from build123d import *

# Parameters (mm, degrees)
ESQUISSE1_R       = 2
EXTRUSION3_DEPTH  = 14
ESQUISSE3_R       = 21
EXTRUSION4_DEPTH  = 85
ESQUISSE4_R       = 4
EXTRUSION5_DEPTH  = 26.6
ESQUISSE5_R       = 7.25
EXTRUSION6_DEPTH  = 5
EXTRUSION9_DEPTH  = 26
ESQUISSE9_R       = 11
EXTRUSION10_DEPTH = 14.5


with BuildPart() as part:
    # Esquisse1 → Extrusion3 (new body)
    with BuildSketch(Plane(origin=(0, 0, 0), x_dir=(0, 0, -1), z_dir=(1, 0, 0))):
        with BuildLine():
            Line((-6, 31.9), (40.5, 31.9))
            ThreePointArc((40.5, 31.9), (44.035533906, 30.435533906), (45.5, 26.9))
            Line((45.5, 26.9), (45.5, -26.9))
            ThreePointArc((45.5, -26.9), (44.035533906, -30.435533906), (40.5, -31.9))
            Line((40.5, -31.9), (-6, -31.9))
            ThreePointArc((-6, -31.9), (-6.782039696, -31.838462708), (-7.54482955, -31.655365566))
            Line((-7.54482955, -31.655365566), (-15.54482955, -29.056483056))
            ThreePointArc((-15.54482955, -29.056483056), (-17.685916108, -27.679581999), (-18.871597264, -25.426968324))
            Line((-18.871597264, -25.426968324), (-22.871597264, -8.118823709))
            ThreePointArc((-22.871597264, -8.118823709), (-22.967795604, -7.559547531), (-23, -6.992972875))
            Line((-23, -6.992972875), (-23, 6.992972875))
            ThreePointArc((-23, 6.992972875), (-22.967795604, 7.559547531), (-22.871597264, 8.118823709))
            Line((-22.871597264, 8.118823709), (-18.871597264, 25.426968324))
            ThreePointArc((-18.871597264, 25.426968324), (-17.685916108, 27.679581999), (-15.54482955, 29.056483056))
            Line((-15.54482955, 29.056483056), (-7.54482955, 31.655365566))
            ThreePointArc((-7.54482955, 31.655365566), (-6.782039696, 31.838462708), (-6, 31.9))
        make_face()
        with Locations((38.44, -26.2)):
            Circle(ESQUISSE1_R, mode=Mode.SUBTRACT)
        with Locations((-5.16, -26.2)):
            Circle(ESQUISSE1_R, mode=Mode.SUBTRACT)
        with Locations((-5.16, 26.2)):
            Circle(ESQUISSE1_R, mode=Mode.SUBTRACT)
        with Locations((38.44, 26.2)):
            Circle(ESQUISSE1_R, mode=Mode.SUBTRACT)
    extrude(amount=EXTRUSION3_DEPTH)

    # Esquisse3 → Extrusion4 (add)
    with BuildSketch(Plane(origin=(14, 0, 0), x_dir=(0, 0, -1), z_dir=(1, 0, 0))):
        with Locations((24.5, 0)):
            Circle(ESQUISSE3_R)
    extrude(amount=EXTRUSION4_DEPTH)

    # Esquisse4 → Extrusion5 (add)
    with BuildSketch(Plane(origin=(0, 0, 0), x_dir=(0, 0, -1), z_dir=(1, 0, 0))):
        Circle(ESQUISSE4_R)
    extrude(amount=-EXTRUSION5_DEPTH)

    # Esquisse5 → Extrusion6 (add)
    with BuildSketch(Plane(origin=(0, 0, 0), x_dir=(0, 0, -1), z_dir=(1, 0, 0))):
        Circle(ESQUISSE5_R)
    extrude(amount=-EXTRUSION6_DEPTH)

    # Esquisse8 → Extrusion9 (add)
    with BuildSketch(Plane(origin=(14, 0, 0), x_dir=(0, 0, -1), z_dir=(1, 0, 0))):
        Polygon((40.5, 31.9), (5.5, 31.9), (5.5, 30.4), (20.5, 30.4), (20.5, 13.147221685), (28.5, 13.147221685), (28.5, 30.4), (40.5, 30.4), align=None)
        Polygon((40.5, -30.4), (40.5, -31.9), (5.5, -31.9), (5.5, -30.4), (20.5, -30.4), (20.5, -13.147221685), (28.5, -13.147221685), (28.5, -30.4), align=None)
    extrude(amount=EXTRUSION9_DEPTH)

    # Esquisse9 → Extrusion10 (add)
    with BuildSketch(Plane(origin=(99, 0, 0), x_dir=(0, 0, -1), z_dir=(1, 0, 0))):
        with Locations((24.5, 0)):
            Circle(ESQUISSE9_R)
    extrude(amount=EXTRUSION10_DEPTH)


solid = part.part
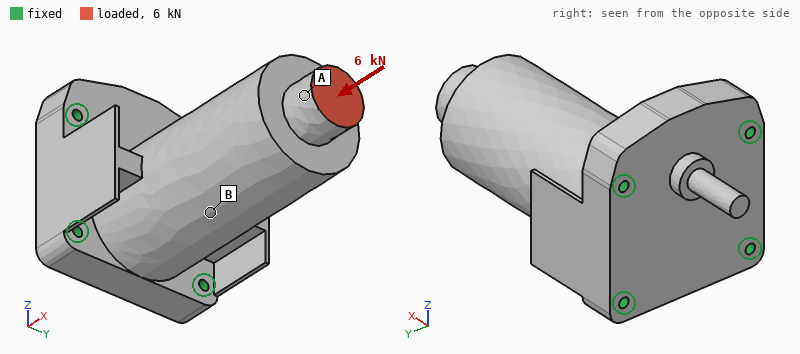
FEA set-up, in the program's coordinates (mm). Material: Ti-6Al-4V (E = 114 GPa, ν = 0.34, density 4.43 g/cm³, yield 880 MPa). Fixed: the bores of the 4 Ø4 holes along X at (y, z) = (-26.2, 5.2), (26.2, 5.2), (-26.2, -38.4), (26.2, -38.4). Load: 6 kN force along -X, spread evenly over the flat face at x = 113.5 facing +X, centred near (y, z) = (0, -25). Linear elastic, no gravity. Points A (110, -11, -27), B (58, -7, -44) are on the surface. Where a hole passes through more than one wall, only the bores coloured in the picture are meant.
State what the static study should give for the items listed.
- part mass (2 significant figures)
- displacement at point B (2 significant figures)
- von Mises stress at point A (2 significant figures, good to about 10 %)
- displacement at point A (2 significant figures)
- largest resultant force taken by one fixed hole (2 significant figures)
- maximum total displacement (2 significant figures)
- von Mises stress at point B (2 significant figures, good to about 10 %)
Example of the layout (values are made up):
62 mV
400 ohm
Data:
840 g
4.6 µm
15 MPa
8.4 µm
2.1 kN
8.9 µm
4.2 MPa
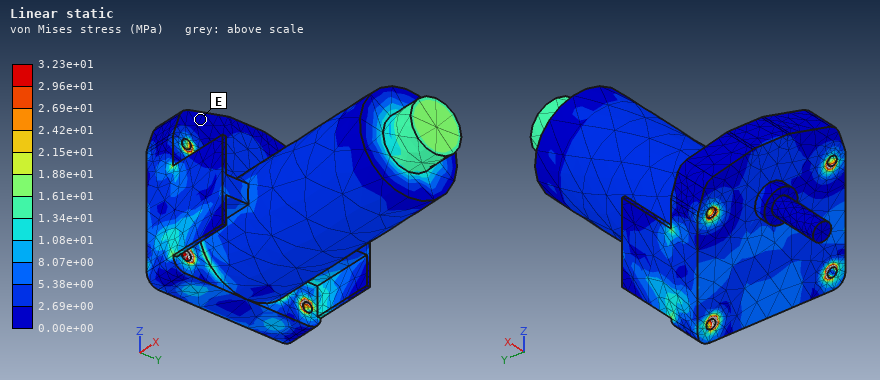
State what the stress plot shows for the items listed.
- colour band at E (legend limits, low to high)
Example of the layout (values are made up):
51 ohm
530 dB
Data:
0.00e+00 to 2.69e+00 MPa
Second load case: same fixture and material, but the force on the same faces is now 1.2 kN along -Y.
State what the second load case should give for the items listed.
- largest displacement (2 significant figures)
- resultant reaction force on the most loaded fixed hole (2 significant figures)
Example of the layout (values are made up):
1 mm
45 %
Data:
34 µm
1.9 kN
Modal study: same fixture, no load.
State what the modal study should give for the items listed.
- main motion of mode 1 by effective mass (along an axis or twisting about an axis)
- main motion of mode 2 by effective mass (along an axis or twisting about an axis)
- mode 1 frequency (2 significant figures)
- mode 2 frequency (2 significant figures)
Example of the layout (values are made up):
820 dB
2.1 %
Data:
along Z
along Y
2200 Hz
2800 Hz
